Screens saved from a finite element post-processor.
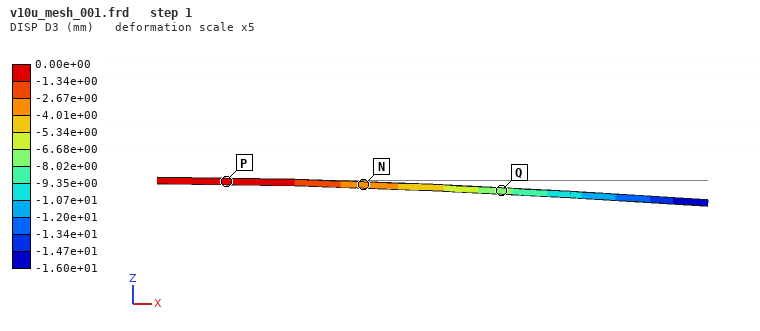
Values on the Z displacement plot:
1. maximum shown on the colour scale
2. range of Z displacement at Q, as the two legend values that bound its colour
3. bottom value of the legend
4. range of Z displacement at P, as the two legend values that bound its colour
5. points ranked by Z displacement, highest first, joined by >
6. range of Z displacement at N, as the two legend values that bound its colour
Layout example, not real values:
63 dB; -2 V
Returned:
0.00e+00 mm; -8.02e+00 to -6.68e+00 mm; -1.60e+01 mm; -1.34e+00 to 0.00e+00 mm; P > N > Q; -4.01e+00 to -2.67e+00 mm
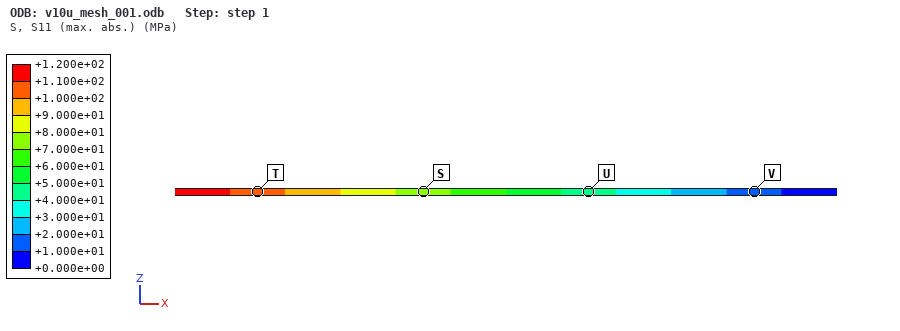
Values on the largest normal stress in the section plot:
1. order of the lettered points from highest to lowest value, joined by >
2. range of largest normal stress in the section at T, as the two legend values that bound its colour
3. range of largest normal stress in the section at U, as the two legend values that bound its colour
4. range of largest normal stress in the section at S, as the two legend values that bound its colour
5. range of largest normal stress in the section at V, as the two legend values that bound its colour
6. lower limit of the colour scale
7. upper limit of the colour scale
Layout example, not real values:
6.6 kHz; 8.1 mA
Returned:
T > S > U > V; +1.000e+02 to +1.100e+02 MPa; +4.000e+01 to +5.000e+01 MPa; +7.000e+01 to +8.000e+01 MPa; +1.000e+01 to +2.000e+01 MPa; +0.000e+00 MPa; +1.200e+02 MPa
